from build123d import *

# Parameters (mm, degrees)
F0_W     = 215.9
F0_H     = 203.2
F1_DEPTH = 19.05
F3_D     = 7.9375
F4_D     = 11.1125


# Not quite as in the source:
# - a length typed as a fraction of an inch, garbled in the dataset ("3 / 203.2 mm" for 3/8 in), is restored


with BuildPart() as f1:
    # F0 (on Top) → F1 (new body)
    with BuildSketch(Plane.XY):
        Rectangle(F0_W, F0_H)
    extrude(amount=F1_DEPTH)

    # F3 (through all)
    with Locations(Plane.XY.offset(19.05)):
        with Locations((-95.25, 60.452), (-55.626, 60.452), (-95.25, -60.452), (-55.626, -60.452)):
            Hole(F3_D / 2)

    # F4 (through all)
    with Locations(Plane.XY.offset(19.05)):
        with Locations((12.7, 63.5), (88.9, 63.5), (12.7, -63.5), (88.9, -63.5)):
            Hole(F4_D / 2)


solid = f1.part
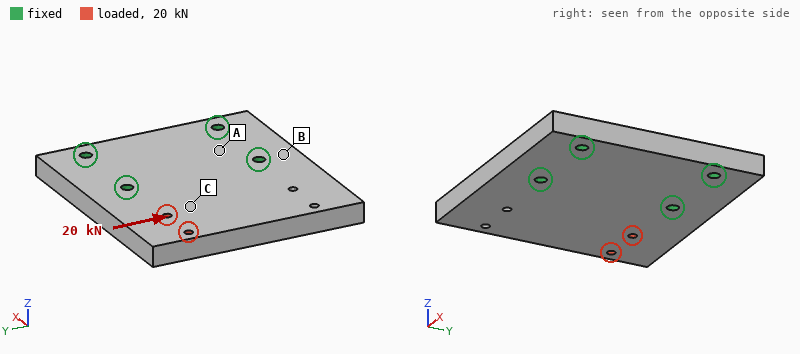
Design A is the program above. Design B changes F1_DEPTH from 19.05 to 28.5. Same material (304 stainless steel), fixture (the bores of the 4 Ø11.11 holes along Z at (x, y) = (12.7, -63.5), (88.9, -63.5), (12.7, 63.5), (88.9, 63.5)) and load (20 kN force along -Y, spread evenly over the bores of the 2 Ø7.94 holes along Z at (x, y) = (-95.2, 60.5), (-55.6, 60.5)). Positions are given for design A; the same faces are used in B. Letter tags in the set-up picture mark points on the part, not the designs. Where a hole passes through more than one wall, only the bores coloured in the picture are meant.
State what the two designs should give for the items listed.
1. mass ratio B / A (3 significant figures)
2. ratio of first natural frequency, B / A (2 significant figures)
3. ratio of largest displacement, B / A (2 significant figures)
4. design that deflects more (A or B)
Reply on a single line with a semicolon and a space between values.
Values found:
1.50; 1.4; 0.67; A
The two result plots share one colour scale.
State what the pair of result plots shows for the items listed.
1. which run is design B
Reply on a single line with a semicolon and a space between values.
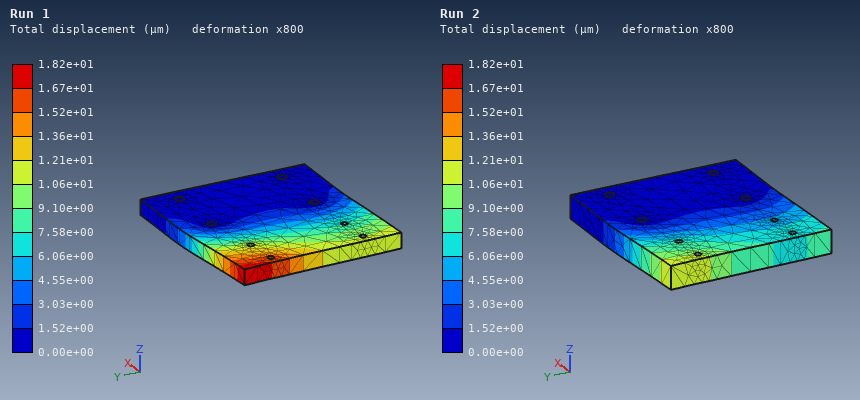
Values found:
Run 2
